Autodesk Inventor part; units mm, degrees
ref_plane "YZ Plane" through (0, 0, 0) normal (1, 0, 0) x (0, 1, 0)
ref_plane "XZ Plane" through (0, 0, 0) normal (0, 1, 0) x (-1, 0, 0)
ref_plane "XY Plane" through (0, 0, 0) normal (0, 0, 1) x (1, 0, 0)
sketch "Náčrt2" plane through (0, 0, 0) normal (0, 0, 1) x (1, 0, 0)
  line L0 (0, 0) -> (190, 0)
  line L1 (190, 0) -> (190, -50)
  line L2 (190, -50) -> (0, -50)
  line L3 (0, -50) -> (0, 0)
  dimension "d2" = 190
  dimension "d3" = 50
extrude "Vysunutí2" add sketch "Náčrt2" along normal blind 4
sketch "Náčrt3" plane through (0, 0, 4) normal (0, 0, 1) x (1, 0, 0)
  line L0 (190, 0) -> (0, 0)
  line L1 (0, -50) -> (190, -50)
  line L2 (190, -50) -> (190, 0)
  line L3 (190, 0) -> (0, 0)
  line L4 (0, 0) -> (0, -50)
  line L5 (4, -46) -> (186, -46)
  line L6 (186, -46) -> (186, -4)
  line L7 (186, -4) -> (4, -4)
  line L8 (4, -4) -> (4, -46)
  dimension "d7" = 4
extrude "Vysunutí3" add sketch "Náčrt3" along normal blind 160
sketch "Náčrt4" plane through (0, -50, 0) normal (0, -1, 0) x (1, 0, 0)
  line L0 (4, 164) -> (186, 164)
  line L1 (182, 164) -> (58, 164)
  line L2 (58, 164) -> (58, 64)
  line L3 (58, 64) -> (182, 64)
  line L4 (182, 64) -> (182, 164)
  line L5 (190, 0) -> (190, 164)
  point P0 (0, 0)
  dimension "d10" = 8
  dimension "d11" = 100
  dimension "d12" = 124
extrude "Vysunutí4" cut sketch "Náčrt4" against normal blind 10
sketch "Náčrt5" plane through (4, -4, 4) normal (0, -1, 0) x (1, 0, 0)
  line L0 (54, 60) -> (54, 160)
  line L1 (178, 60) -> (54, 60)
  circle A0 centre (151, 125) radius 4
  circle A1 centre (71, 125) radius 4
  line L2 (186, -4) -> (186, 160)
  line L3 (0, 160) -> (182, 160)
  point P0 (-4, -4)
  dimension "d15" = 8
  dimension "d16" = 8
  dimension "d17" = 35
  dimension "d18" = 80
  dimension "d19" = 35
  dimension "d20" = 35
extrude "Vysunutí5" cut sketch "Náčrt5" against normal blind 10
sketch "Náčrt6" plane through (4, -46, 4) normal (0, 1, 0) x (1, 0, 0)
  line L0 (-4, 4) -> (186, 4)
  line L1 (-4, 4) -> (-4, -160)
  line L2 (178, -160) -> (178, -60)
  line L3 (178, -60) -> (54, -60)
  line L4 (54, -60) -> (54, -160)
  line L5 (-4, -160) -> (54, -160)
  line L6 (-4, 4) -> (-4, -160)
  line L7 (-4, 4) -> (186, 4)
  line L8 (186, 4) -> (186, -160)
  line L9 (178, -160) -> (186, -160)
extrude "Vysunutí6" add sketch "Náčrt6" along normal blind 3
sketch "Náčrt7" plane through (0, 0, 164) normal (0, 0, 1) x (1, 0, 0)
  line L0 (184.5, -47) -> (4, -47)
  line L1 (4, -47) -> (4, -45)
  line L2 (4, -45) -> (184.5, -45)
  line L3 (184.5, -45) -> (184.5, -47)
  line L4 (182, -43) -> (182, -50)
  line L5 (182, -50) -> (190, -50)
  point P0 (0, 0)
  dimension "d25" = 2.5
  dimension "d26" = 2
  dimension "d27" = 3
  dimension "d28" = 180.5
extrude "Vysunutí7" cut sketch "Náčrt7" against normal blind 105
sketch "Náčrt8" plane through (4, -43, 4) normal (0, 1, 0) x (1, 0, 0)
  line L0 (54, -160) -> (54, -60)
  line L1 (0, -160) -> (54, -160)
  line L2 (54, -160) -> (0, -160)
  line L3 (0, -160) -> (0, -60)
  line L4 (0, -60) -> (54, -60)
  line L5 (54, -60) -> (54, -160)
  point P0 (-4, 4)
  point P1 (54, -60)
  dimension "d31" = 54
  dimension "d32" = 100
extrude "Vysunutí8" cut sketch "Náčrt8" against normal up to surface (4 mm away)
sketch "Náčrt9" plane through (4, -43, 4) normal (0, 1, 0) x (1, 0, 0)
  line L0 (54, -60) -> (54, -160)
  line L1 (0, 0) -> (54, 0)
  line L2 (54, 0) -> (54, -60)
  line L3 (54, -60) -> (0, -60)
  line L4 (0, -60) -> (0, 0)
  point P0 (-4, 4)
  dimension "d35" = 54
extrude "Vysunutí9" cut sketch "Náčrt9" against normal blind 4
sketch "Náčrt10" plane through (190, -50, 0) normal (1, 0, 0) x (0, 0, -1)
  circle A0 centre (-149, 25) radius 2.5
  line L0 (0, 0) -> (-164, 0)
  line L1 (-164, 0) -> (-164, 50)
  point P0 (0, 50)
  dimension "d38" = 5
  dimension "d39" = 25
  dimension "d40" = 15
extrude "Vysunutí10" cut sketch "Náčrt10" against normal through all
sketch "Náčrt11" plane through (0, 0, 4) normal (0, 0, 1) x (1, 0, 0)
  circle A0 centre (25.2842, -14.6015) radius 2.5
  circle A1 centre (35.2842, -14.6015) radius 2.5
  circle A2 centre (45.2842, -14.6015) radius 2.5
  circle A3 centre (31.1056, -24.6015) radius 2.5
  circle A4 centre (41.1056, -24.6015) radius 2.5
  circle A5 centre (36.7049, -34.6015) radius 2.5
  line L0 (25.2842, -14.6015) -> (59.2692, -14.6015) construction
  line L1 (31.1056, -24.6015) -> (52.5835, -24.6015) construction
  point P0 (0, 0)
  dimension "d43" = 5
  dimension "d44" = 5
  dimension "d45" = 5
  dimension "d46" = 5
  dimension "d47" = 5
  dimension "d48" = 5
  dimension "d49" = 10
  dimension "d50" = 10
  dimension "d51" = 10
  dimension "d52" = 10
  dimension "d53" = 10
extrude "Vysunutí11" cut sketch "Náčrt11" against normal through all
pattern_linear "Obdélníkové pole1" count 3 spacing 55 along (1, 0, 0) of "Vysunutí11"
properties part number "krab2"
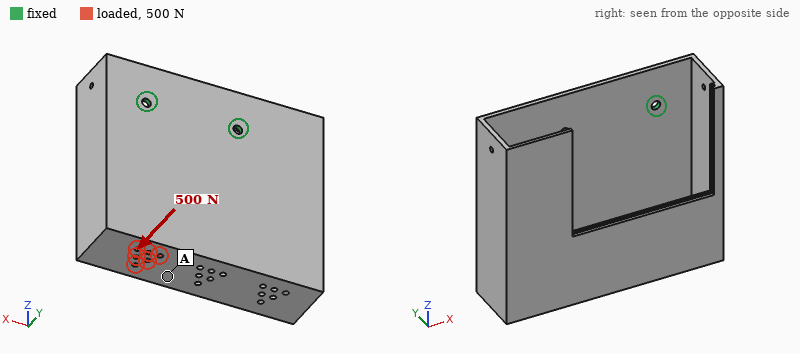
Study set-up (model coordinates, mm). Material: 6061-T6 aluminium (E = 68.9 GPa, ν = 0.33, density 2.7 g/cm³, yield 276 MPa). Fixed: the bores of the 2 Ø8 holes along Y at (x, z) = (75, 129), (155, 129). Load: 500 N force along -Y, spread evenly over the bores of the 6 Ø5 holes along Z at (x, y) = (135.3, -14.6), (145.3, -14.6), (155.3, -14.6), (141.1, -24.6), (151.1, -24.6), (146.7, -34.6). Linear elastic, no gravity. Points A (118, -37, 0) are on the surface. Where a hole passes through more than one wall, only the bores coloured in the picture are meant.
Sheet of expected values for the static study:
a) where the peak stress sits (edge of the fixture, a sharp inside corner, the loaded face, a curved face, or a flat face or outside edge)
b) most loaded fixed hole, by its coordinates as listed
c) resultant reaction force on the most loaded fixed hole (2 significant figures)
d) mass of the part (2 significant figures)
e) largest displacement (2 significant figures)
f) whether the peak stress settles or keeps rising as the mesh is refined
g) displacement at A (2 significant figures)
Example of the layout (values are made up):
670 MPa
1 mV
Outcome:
edge of the fixture
(155, 129)
380 N
800 g
3.0 mm
keeps rising
2.7 mm
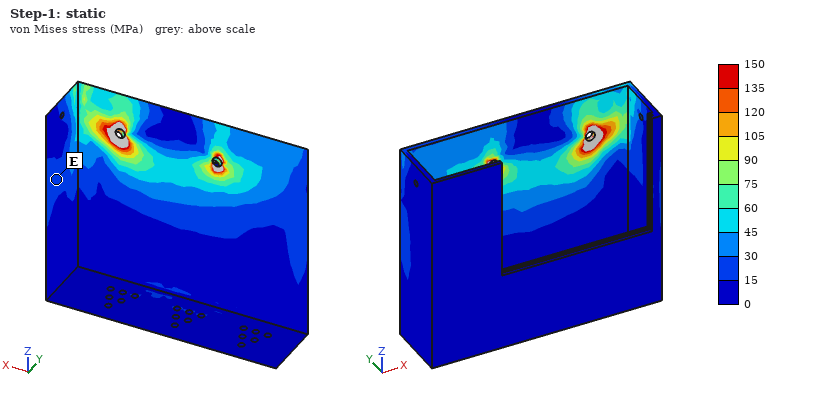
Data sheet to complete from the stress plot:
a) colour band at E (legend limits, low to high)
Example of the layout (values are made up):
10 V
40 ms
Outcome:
15 to 30 MPa
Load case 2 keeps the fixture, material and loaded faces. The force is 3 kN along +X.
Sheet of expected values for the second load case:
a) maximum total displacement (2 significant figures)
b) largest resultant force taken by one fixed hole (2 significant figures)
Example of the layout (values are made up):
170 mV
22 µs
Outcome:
1.6 mm
4.8 kN
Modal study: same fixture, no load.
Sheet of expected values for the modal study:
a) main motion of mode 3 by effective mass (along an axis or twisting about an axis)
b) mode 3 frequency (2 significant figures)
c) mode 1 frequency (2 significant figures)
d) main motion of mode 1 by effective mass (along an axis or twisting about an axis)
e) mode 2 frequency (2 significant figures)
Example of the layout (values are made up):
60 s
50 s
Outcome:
along Y
440 Hz
120 Hz
along Y
200 Hz
